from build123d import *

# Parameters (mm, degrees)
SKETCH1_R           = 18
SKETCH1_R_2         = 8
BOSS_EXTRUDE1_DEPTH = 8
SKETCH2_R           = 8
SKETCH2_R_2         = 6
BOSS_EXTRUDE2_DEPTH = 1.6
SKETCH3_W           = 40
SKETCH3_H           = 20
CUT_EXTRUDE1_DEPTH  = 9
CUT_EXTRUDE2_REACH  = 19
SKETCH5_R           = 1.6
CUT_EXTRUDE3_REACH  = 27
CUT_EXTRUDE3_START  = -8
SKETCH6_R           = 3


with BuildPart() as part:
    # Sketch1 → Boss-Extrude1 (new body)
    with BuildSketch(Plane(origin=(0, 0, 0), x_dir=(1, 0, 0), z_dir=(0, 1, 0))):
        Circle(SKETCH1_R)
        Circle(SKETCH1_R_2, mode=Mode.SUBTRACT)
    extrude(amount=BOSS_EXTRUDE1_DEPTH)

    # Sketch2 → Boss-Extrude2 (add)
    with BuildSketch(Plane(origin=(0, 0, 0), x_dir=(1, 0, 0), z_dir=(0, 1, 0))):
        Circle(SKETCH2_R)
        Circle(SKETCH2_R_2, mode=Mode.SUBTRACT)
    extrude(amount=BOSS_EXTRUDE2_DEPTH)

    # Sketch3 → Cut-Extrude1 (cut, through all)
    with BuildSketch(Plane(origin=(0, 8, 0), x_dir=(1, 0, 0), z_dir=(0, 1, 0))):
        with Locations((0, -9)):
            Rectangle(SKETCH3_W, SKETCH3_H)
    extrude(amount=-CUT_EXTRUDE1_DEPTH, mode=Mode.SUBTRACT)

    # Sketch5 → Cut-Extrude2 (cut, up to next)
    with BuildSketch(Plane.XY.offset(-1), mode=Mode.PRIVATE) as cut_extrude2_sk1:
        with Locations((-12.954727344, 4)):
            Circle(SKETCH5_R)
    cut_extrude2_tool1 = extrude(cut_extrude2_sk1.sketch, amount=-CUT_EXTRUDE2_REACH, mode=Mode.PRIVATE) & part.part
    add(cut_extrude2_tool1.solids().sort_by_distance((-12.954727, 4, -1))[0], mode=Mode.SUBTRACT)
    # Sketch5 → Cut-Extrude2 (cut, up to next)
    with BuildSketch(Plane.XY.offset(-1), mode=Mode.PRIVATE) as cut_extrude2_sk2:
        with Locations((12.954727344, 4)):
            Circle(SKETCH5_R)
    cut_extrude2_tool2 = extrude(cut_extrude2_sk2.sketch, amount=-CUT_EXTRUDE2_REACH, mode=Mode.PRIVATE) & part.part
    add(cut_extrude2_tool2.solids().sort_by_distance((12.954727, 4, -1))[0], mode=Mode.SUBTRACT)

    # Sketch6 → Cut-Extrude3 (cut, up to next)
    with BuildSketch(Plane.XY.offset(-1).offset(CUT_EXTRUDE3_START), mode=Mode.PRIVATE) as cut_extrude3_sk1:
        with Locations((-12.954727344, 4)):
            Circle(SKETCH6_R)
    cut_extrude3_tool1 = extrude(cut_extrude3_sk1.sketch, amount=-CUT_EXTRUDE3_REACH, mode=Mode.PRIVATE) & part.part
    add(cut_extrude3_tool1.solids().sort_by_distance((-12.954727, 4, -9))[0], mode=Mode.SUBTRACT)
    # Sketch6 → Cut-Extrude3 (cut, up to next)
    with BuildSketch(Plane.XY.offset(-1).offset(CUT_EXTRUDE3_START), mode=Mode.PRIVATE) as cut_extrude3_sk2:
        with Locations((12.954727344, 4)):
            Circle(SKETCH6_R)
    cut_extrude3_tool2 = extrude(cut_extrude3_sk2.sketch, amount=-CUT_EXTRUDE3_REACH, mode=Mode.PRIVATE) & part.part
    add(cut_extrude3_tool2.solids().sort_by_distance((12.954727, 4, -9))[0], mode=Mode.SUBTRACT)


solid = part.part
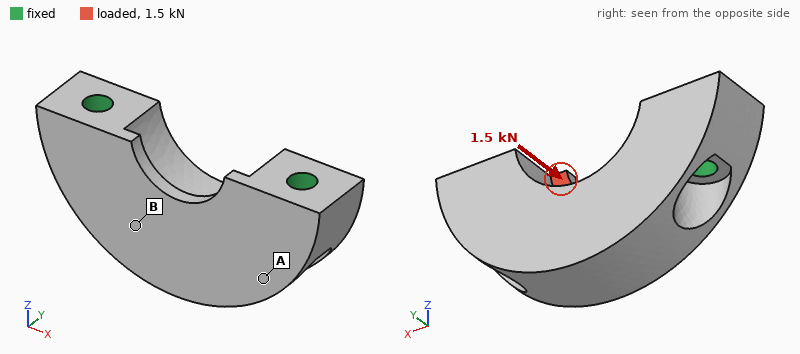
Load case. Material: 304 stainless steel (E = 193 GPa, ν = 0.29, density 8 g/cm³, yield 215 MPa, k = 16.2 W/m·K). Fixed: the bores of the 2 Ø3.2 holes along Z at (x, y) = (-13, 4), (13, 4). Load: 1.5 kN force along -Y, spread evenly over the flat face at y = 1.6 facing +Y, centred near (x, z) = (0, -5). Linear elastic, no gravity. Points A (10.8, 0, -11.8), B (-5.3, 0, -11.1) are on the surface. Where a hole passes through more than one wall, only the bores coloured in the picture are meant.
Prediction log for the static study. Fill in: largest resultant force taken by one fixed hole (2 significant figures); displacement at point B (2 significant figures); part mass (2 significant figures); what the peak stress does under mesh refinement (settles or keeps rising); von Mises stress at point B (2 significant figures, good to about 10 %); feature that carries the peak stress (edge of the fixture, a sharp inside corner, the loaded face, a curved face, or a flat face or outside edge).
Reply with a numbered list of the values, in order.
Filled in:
1. 760 N
2. 2.0 µm
3. 23 g
4. keeps rising
5. 26 MPa
6. a sharp inside corner
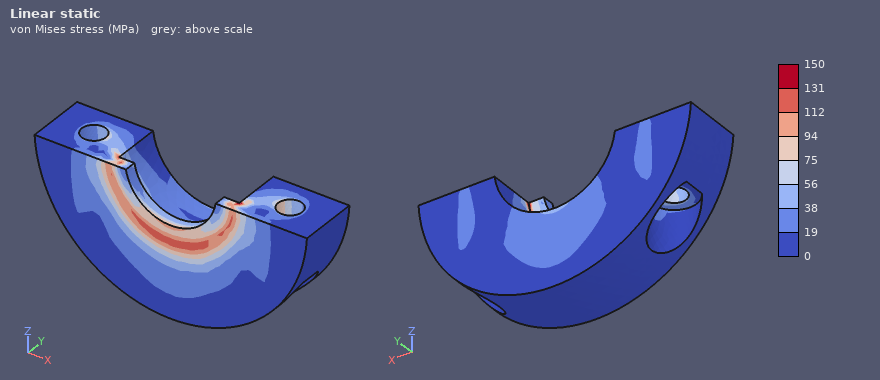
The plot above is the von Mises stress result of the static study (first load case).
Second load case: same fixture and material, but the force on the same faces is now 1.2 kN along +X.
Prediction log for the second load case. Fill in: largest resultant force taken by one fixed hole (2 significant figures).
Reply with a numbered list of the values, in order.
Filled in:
1. 600 N
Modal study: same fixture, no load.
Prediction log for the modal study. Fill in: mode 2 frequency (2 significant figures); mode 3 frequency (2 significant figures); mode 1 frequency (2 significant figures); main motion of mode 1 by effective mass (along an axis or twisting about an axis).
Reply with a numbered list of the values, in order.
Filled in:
1. 47 kHz
2. 49 kHz
3. 21 kHz
4. along Y
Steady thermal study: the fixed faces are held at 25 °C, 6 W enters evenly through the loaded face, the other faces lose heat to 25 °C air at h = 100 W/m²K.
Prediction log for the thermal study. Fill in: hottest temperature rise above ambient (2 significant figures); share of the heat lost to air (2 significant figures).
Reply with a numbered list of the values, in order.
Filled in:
1. 41 K
2. 22 %
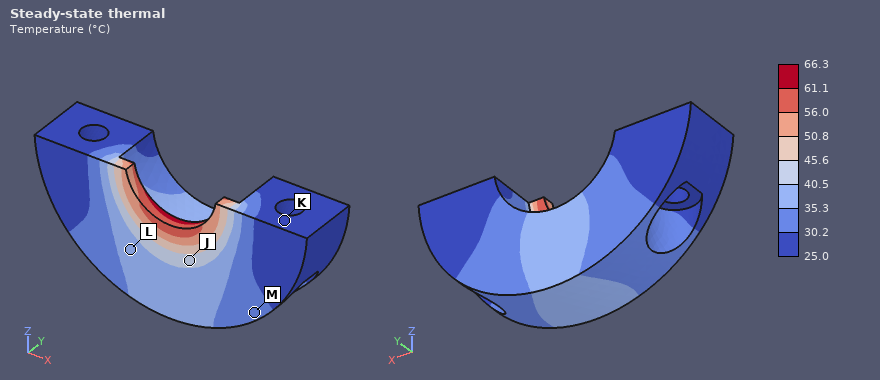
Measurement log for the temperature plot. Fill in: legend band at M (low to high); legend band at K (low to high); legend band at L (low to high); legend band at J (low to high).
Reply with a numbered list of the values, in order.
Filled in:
1. 30.2 to 35.3 °C
2. 25.0 to 30.2 °C
3. 35.3 to 40.5 °C
4. 40.5 to 45.6 °C
